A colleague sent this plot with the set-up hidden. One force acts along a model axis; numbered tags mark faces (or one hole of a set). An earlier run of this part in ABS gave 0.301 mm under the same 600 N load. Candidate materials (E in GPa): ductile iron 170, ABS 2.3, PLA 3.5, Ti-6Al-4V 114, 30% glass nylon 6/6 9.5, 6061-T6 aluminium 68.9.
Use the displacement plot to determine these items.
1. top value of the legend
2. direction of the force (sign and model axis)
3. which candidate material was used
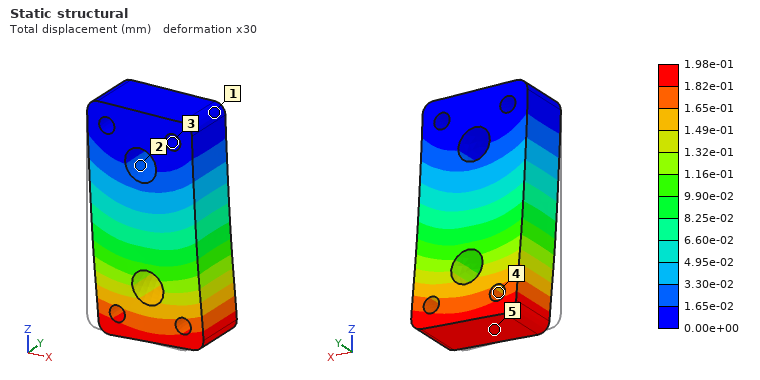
1.98e-01 mm
+X
PLA
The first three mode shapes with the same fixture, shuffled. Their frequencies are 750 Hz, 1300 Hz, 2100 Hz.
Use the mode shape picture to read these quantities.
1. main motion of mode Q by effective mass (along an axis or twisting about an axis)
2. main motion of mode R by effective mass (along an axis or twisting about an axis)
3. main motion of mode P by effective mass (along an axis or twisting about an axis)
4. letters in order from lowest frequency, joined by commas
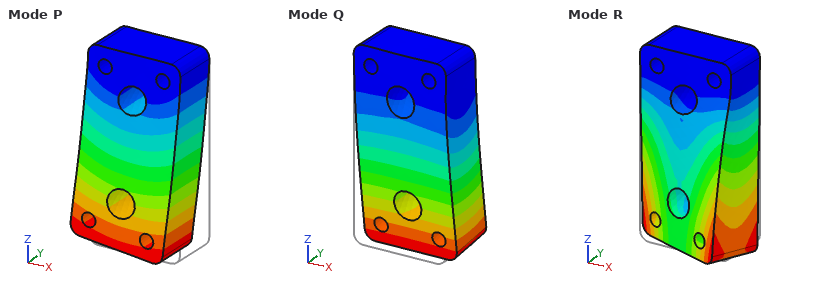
along Y
twisting about Z
along X
Q, P, R
